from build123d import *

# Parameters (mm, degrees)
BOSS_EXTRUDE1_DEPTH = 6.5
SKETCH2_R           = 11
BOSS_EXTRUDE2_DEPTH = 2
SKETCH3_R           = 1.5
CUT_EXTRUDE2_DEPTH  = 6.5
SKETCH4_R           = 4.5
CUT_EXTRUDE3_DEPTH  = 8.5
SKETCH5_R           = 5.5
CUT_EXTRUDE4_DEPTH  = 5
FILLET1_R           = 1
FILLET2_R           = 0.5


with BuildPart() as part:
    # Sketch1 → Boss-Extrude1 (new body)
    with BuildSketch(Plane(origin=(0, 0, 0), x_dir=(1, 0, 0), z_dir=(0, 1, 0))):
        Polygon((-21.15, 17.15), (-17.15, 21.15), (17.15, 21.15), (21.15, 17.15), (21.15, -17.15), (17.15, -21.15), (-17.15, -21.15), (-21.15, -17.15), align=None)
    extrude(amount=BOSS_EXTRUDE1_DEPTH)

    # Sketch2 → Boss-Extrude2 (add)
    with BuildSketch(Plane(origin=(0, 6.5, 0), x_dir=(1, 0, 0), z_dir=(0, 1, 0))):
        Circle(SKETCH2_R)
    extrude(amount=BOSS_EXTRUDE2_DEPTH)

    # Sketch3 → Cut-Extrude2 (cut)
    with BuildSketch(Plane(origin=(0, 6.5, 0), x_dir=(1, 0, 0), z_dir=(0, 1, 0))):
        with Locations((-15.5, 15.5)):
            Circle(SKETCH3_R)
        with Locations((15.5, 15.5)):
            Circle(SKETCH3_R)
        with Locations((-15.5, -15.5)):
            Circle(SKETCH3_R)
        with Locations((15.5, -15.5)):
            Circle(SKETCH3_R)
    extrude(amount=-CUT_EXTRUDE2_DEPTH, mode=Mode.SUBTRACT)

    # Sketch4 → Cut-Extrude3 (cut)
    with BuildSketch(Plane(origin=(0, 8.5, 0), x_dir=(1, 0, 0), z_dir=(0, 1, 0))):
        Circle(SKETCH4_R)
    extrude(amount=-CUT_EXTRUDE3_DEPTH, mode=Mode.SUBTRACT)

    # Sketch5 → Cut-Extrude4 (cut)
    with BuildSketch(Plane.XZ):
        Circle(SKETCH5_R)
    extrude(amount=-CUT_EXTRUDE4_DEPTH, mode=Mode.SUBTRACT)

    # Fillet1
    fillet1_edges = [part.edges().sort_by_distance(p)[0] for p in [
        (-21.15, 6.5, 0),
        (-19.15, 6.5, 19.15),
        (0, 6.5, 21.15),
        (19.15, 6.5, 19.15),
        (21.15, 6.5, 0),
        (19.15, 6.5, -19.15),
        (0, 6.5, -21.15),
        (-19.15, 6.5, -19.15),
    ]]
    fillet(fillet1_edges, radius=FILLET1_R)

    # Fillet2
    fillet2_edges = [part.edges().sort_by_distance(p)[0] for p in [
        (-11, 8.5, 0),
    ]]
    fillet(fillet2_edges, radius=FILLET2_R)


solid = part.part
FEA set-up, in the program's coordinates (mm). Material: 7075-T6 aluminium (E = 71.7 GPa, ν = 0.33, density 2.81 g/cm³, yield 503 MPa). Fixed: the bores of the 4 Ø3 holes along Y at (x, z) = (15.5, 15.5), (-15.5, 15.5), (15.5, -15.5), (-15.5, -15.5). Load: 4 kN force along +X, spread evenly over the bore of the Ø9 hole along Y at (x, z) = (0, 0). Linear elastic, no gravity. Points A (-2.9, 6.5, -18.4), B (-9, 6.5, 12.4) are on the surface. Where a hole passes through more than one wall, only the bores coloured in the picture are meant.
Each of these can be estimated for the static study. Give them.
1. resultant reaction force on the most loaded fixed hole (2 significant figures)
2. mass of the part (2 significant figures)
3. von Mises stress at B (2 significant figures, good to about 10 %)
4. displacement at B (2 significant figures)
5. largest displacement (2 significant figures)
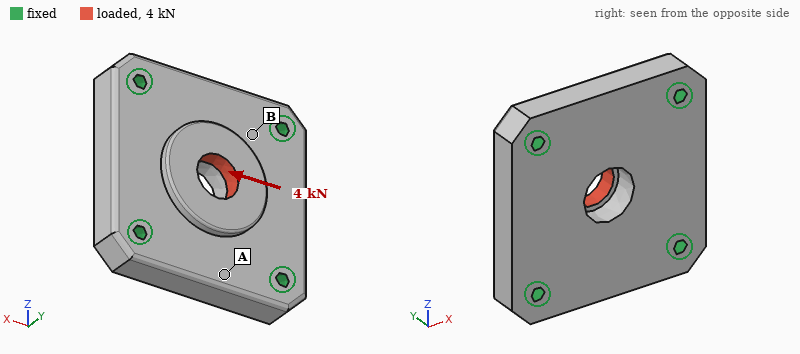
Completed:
1.1 kN
32 g
21 MPa
1.9 µm
9.5 µm
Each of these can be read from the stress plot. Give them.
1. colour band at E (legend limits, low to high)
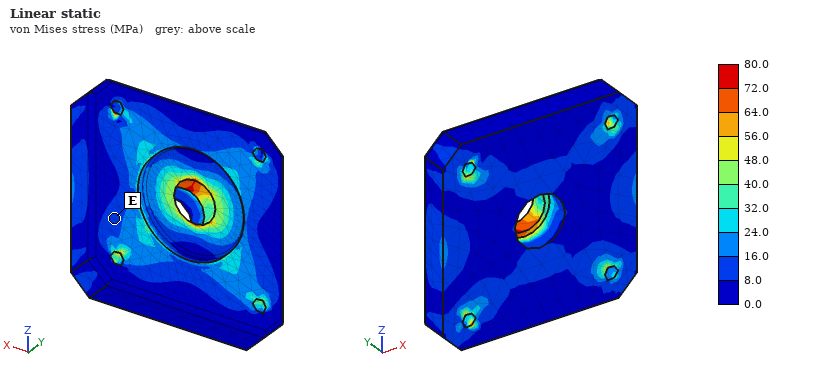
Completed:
8.0 to 16.0 MPa
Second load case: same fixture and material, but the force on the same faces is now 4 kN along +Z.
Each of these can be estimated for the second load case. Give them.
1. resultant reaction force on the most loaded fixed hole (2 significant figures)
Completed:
1.1 kN
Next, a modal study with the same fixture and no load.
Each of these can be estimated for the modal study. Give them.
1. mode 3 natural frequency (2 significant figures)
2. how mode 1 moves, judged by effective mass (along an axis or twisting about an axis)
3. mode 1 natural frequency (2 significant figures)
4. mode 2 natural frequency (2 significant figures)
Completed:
29 kHz
along Y
21 kHz
29 kHz
